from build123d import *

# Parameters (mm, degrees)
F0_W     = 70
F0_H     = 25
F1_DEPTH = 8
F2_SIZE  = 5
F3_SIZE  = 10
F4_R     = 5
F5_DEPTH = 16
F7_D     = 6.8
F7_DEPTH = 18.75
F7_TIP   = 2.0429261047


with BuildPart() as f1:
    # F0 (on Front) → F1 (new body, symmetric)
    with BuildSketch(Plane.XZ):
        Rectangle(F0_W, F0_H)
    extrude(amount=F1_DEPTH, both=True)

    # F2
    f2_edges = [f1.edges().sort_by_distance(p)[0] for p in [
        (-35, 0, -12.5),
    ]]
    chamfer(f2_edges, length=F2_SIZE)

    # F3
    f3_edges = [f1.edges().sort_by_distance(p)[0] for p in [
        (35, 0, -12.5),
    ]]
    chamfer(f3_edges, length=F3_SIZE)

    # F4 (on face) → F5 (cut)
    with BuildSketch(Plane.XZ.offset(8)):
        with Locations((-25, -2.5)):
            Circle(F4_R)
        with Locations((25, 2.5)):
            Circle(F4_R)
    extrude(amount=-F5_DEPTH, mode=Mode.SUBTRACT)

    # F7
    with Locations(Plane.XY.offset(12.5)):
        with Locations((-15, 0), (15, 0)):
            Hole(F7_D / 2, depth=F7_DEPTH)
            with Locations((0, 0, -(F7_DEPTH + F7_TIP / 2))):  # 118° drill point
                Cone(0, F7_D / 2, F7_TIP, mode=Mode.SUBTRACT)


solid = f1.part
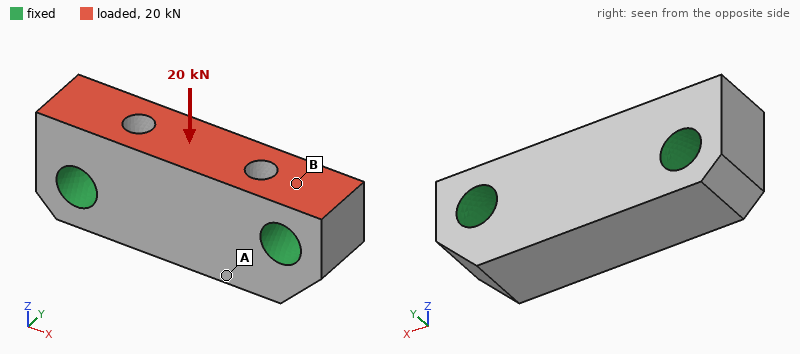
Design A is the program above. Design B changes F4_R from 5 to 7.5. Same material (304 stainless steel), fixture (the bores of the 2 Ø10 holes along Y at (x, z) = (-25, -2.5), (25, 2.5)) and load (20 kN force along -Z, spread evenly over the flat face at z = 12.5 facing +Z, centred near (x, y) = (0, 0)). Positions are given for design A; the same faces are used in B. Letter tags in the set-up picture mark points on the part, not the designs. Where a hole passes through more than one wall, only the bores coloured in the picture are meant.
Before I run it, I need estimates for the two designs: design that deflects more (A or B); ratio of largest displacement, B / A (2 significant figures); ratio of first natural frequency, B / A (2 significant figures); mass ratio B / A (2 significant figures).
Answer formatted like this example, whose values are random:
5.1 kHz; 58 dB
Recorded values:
A; 0.77; 1.2; 0.86
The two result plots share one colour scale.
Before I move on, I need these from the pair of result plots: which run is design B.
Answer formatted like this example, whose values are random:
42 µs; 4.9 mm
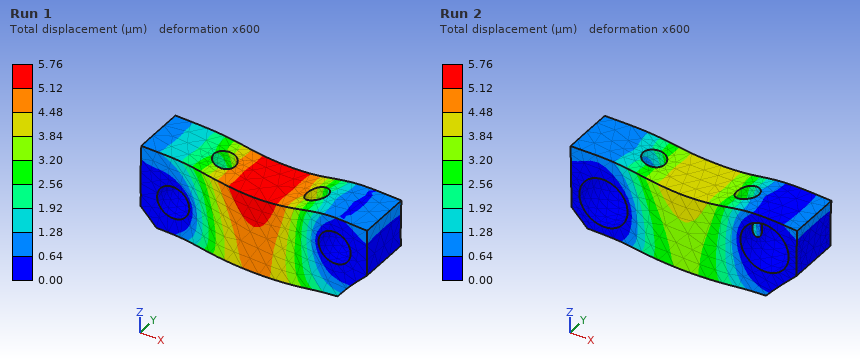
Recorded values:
Run 2
